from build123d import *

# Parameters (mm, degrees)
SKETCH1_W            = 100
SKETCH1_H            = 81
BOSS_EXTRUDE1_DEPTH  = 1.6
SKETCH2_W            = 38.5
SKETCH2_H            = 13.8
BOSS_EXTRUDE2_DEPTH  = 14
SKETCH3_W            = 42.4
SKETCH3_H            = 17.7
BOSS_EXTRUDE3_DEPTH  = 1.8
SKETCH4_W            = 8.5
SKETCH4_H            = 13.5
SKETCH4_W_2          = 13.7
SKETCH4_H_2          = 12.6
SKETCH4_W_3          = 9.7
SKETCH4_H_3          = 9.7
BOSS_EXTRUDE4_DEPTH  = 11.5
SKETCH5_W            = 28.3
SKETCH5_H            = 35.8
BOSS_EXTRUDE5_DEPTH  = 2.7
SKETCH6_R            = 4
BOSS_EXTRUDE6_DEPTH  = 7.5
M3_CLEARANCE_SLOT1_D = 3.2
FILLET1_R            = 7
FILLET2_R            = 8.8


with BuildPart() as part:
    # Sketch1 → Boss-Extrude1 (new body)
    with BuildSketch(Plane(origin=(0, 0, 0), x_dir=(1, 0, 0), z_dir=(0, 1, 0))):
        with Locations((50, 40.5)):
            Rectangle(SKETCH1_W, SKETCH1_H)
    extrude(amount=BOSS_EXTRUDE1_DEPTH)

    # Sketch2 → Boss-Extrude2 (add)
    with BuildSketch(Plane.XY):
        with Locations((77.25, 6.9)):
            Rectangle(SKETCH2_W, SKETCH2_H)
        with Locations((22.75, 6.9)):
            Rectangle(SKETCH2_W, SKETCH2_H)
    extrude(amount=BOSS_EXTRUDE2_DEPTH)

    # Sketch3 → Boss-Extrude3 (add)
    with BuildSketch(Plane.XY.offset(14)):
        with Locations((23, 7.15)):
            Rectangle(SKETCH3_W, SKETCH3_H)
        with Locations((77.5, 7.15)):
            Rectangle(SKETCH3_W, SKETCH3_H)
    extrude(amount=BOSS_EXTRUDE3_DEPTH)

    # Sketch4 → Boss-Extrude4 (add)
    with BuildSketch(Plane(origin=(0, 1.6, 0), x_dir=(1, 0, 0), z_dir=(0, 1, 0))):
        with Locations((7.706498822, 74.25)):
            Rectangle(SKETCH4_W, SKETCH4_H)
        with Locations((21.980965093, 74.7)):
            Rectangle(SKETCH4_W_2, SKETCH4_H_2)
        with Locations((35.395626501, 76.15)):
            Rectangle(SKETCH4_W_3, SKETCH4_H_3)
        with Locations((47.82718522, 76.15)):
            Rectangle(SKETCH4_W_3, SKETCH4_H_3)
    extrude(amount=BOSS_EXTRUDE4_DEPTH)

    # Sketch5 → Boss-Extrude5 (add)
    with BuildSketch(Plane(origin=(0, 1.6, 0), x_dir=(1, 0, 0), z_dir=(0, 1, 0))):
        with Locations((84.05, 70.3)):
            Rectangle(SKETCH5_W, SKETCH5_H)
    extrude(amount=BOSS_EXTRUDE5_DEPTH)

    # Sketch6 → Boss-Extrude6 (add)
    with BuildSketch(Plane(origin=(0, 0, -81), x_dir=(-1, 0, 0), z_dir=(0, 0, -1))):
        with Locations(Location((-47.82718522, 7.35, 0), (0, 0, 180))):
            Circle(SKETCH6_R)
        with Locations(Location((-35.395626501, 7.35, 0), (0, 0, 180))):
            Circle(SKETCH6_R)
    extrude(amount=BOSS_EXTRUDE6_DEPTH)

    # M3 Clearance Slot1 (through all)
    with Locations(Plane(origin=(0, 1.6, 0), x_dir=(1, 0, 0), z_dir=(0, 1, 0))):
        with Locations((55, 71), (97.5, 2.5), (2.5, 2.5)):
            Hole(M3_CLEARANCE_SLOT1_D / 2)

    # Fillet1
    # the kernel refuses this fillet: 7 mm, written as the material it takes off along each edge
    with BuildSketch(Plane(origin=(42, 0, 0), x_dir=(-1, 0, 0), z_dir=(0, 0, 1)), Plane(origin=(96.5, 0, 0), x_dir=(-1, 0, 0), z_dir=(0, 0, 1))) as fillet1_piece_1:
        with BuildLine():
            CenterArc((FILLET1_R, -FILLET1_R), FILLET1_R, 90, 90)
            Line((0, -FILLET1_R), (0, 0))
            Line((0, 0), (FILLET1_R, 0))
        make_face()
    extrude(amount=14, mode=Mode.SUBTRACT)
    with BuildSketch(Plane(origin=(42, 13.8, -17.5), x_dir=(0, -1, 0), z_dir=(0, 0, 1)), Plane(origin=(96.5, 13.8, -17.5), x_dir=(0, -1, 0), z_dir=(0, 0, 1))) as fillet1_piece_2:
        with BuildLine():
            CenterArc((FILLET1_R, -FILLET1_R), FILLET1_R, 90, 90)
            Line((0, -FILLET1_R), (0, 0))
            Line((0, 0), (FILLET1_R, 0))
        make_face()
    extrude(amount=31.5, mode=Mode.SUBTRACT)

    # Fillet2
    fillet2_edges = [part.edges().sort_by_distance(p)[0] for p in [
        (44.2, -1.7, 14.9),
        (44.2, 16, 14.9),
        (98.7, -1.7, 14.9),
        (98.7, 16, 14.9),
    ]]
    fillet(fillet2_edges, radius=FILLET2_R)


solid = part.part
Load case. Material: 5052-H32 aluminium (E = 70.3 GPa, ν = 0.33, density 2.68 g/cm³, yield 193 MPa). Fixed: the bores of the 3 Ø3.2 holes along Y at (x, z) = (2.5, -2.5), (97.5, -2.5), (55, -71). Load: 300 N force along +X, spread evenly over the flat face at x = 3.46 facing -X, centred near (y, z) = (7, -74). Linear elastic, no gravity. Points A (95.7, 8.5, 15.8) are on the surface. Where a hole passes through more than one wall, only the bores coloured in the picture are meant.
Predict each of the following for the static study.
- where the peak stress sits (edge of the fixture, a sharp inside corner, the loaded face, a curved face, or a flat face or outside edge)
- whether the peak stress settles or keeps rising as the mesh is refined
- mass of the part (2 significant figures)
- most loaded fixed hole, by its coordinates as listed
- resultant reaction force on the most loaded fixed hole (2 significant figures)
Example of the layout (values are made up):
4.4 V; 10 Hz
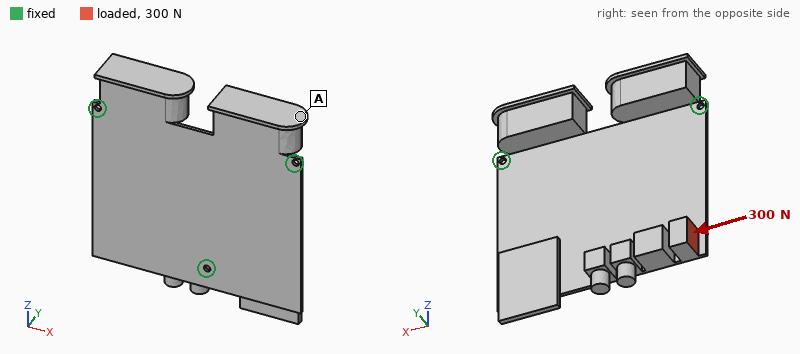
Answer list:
edge of the fixture; keeps rising; 100 g; (55, -71); 280 N
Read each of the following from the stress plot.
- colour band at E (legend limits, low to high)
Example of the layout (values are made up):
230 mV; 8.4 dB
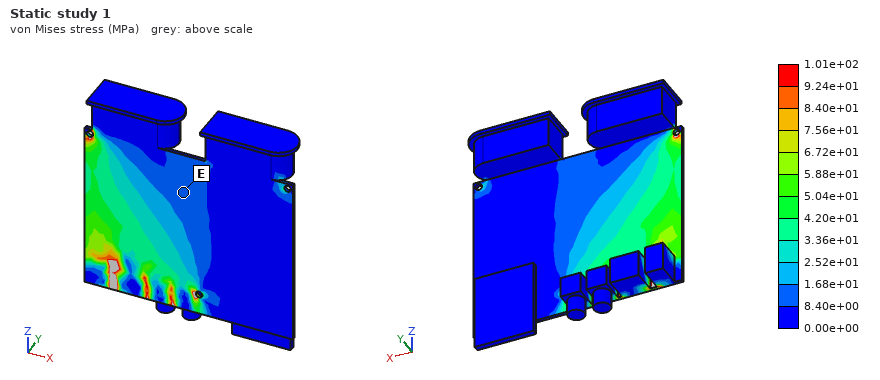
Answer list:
8.40e+00 to 1.68e+01 MPa
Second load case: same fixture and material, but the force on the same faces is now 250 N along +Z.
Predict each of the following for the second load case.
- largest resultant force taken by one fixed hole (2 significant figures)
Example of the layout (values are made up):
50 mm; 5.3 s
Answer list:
140 N
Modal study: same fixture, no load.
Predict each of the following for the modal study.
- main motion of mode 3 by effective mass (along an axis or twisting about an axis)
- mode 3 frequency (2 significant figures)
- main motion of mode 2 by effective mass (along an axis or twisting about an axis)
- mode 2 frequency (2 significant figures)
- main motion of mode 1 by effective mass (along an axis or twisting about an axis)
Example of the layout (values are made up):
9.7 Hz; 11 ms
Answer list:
along Y; 620 Hz; along Y; 430 Hz; twisting about X
